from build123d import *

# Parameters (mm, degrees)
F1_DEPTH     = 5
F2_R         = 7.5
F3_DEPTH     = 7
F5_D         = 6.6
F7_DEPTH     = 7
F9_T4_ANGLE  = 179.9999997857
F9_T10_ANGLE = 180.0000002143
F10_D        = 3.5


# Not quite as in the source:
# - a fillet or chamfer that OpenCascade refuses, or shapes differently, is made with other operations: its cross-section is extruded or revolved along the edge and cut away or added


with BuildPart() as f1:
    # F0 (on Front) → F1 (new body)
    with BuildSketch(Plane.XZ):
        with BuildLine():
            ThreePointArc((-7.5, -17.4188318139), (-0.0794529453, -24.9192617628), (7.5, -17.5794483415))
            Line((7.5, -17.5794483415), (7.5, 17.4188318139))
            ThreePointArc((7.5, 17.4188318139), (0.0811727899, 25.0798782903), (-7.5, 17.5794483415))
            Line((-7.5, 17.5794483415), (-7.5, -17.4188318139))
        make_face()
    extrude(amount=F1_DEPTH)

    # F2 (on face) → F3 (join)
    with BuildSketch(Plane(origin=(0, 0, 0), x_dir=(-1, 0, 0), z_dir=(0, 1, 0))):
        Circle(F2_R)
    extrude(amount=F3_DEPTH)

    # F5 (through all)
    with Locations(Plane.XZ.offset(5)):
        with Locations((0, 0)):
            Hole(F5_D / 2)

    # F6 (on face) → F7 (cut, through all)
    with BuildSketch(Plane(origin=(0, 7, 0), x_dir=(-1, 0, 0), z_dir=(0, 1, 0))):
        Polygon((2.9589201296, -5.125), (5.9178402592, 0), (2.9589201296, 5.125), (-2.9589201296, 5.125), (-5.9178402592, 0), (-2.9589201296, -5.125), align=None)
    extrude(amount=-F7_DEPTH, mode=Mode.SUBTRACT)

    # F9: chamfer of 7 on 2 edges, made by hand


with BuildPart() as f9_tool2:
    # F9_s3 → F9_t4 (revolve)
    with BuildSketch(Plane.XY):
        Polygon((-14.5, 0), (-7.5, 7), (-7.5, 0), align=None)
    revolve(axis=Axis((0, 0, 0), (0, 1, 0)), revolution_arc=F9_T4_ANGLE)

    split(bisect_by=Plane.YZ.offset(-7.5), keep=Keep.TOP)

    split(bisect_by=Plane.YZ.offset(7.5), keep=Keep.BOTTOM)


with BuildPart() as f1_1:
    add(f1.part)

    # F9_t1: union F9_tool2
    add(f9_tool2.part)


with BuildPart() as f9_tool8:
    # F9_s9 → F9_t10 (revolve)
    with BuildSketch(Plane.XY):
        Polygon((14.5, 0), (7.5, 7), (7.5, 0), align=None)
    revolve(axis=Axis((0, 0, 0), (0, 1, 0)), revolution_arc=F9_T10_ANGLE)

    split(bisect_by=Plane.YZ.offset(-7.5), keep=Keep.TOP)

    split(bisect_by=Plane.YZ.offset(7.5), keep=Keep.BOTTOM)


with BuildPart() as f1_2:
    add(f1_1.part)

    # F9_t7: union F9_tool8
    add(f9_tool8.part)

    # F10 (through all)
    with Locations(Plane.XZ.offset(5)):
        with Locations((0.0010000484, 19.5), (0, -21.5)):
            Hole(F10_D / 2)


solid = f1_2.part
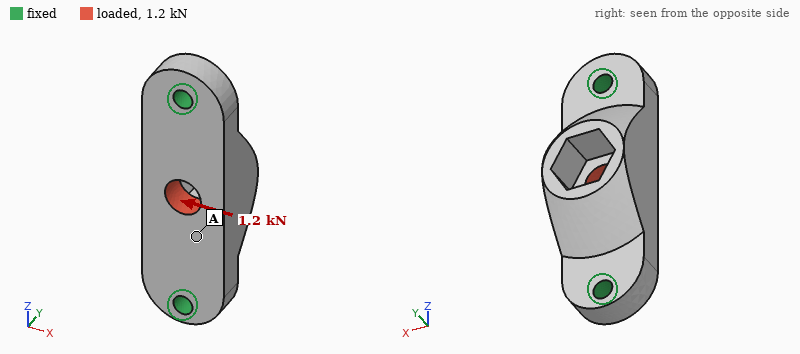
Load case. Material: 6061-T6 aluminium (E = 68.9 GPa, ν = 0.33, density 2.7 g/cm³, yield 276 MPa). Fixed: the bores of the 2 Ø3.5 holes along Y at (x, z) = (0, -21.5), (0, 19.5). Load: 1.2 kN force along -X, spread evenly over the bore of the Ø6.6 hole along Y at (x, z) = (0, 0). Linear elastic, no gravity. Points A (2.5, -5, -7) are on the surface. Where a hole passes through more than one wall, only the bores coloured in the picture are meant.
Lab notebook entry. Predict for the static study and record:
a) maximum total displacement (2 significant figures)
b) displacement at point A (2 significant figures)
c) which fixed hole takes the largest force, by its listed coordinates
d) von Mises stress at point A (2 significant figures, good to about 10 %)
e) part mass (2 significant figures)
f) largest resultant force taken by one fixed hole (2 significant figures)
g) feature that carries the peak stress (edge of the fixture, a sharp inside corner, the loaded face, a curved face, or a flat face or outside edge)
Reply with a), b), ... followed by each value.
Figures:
a) 13 µm
b) 11 µm
c) (0, 19.5)
d) 12 MPa
e) 13 g
f) 630 N
g) edge of the fixture
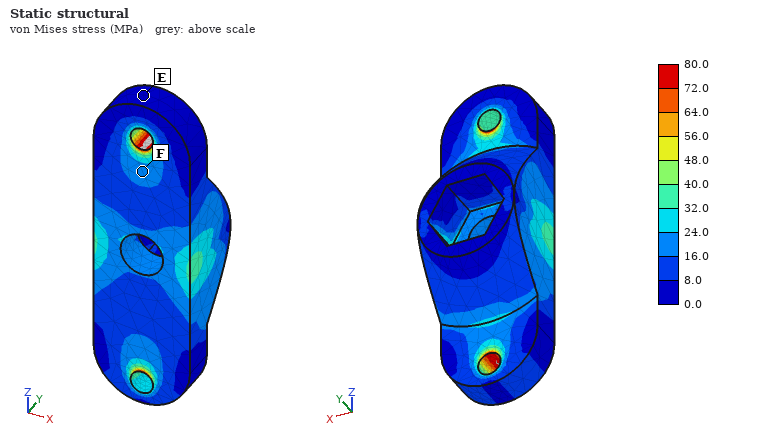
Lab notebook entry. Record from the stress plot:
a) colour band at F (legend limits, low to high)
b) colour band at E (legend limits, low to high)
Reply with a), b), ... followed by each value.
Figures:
a) 16.0 to 24.0 MPa
b) 0.0 to 8.0 MPa
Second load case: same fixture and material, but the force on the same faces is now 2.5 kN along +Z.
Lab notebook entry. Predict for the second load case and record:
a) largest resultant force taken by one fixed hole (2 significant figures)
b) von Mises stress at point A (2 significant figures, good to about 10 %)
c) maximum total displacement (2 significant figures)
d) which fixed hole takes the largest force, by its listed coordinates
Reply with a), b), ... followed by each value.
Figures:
a) 1.3 kN
b) 24 MPa
c) 6.1 µm
d) (0, 19.5)
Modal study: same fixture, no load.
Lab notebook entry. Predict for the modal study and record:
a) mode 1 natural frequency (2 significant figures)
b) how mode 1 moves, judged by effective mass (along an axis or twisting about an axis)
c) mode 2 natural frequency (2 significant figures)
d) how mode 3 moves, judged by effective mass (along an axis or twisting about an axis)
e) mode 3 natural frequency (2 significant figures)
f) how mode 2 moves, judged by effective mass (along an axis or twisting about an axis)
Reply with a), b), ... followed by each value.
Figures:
a) 14 kHz
b) along X
c) 15 kHz
d) along X
e) 23 kHz
f) along Y
